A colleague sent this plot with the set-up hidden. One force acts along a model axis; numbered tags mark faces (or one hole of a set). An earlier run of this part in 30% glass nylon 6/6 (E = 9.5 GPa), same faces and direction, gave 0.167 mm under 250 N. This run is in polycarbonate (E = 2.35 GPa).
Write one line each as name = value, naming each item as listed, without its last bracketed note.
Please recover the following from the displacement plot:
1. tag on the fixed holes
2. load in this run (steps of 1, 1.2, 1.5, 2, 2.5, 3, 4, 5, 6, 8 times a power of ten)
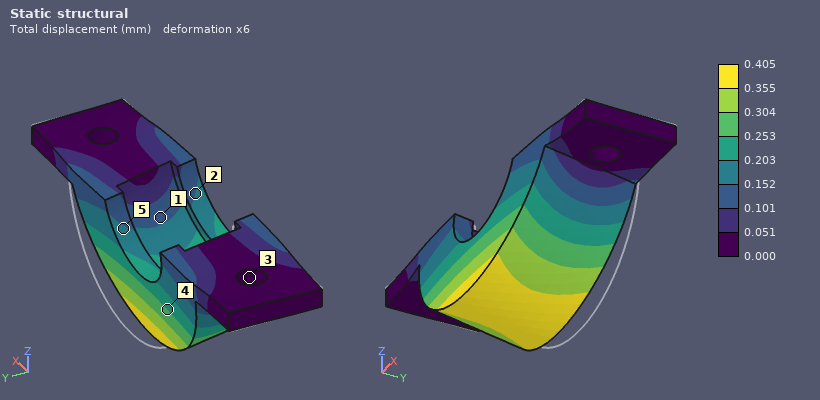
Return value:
tag on the fixed holes = 3
load in this run = 150 N
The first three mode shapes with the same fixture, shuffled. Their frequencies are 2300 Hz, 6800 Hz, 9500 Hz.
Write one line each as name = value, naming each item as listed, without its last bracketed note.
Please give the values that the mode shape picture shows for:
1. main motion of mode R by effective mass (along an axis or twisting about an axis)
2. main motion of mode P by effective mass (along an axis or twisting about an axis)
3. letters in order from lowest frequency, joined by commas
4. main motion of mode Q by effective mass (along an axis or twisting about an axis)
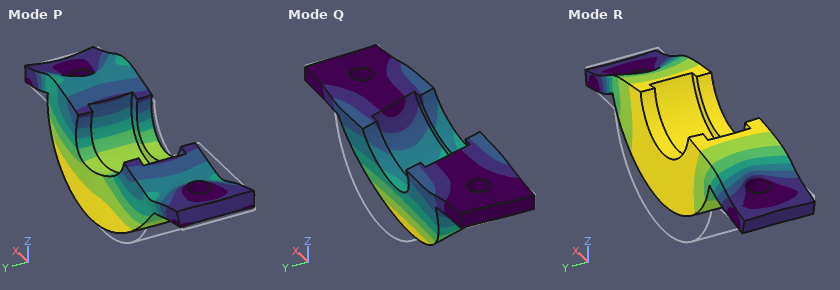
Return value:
main motion of mode R by effective mass = along Z
main motion of mode P by effective mass = along X
letters in order from lowest frequency, joined by commas = Q, R, P
main motion of mode Q by effective mass = along Y
